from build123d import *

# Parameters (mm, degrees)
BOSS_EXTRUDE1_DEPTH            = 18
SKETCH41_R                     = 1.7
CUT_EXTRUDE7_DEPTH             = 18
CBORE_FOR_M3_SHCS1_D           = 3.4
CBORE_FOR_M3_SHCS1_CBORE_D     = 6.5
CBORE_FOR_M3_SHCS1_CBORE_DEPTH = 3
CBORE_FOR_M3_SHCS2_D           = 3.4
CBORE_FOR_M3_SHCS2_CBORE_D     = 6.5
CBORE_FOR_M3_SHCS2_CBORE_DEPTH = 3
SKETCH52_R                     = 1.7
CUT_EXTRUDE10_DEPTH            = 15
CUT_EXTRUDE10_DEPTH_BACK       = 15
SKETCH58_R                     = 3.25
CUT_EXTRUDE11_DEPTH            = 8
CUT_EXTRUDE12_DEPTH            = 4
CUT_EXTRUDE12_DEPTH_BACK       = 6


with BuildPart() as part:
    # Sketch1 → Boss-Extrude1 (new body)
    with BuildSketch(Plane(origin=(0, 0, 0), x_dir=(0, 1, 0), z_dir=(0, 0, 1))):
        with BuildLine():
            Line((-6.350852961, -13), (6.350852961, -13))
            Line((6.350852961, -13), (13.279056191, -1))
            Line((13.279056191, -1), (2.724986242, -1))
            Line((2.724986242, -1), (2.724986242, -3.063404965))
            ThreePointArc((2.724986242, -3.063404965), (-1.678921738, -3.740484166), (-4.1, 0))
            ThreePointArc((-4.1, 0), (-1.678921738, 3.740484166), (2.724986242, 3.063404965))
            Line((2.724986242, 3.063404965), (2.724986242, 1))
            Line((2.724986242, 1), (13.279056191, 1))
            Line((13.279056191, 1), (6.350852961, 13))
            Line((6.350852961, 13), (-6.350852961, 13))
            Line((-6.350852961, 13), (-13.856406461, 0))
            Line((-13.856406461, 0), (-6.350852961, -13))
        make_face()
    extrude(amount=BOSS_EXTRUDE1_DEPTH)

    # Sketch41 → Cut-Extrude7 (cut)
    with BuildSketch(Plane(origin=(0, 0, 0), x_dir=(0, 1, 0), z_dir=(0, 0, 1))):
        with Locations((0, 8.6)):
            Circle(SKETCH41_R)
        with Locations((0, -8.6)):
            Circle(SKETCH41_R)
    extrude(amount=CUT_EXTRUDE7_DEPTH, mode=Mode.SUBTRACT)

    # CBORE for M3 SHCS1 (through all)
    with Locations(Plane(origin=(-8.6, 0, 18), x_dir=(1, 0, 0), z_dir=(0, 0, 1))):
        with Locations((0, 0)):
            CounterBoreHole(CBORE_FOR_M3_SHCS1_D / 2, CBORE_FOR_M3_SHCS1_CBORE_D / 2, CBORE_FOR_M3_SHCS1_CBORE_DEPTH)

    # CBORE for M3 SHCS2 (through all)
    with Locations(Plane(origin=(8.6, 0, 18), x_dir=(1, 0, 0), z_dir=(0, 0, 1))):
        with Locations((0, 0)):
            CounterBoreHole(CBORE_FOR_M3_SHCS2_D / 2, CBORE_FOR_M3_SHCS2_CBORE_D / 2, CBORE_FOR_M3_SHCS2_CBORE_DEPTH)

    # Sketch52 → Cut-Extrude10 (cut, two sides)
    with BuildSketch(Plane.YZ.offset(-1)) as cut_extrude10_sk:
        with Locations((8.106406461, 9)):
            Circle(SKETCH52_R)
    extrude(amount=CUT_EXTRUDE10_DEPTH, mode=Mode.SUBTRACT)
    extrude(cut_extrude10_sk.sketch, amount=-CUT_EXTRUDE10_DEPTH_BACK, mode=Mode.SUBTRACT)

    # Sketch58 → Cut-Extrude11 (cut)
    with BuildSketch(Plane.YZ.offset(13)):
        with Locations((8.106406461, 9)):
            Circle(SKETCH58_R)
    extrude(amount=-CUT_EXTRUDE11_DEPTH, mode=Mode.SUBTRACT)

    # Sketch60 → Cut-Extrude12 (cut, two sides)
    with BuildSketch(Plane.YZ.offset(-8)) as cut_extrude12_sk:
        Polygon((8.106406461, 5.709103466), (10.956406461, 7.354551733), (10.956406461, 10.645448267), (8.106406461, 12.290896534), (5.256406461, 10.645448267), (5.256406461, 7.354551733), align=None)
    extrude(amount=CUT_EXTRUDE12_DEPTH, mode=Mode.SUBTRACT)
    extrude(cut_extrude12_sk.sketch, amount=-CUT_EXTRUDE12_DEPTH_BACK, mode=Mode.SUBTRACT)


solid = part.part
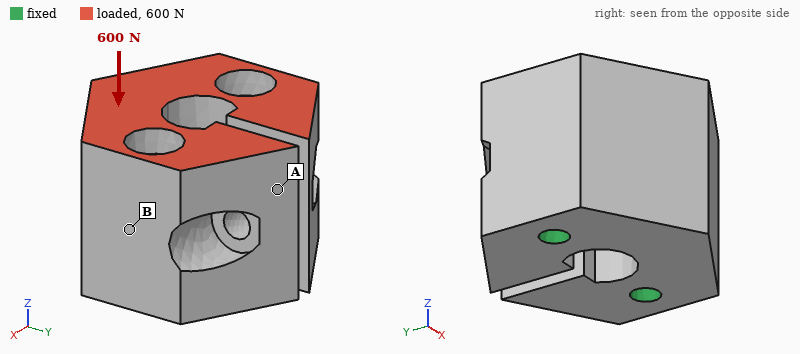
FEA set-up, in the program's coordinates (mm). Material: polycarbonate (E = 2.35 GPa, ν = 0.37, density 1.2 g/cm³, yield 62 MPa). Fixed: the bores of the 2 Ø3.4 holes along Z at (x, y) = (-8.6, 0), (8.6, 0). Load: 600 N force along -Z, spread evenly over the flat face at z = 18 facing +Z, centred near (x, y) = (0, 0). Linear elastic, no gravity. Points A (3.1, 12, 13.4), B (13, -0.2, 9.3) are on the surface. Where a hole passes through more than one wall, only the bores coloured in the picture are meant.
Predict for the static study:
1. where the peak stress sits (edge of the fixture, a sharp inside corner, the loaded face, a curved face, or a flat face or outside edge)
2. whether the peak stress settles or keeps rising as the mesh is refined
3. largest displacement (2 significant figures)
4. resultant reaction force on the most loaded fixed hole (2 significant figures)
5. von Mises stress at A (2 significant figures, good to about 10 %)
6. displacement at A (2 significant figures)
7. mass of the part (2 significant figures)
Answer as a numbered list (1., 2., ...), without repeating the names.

1. edge of the fixture
2. keeps rising
3. 31 µm
4. 300 N
5. 2.2 MPa
6. 23 µm
7. 8.8 g
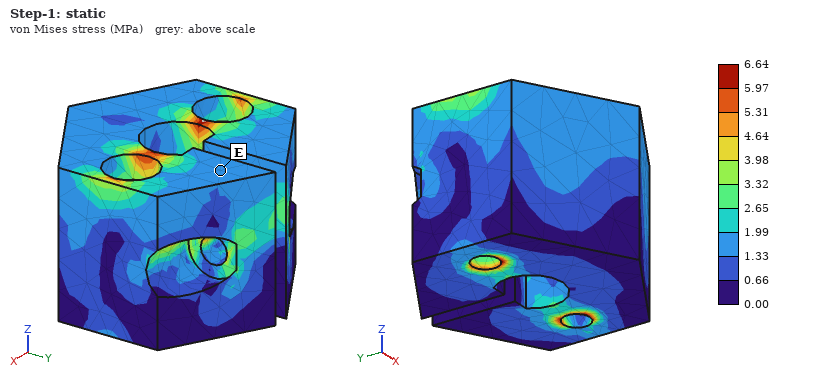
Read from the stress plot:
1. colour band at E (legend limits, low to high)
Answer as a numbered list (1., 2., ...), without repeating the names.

1. 1.33 to 1.99 MPa
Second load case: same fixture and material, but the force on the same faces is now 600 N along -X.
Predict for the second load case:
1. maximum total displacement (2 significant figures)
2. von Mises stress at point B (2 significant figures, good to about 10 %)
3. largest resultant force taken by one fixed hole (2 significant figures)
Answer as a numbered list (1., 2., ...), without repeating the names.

1. 92 µm
2. 4.0 MPa
3. 320 N
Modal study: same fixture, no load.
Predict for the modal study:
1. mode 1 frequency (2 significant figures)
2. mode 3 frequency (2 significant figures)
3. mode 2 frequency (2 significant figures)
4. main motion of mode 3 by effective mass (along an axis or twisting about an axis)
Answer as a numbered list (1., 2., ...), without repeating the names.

1. 8900 Hz
2. 11 kHz
3. 9000 Hz
4. twisting about X
